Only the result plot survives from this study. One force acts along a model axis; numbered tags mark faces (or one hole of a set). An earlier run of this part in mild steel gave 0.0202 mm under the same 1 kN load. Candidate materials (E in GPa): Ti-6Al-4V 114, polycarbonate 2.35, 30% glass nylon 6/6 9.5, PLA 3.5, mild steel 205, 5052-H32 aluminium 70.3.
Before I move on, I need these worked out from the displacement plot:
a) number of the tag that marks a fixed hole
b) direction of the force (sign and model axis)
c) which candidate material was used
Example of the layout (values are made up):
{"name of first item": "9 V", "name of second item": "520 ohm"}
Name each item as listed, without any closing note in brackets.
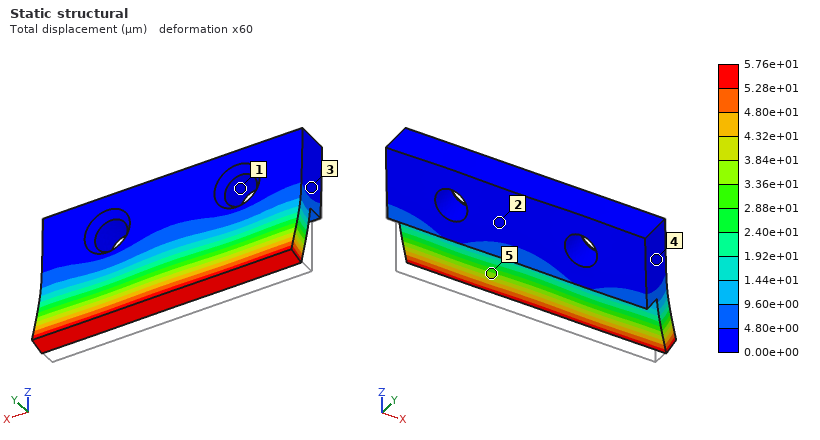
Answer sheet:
{"number of the tag that marks a fixed hole": "1", "direction of the force": "+Y", "which candidate material was used": "5052-H32 aluminium"}
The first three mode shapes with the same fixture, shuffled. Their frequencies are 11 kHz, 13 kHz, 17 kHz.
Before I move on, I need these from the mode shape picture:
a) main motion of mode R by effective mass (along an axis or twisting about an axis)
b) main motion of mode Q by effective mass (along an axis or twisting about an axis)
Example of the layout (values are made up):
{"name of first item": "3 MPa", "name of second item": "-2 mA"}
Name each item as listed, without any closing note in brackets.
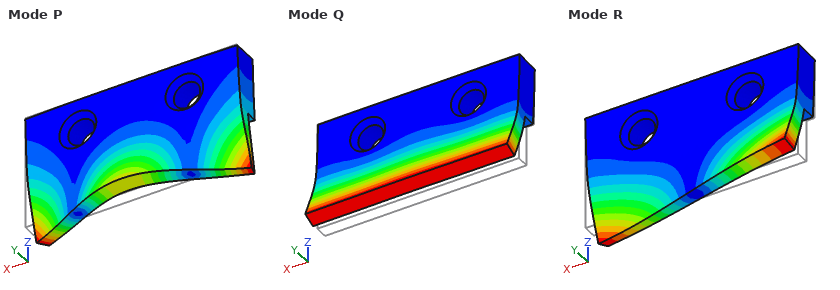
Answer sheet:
{"main motion of mode R by effective mass": "twisting about Z", "main motion of mode Q by effective mass": "along Y"}
